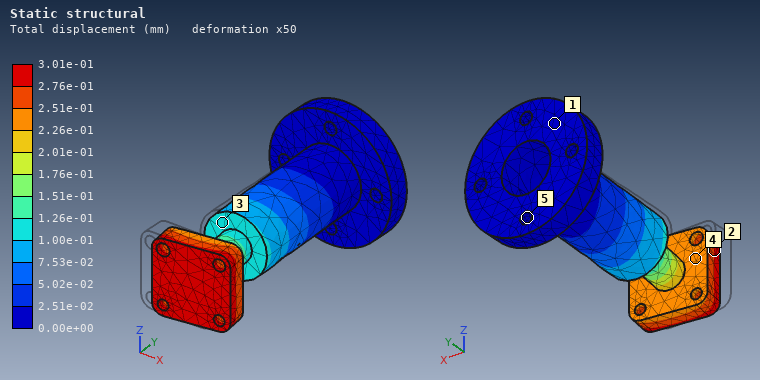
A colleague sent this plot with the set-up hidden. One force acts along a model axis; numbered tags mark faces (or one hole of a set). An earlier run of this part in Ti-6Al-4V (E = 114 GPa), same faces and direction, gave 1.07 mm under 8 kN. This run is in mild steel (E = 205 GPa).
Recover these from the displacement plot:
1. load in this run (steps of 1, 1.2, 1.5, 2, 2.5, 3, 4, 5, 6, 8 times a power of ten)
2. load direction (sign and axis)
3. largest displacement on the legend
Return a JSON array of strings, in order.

["4 kN", "+X", "3.01e-01 mm"]
